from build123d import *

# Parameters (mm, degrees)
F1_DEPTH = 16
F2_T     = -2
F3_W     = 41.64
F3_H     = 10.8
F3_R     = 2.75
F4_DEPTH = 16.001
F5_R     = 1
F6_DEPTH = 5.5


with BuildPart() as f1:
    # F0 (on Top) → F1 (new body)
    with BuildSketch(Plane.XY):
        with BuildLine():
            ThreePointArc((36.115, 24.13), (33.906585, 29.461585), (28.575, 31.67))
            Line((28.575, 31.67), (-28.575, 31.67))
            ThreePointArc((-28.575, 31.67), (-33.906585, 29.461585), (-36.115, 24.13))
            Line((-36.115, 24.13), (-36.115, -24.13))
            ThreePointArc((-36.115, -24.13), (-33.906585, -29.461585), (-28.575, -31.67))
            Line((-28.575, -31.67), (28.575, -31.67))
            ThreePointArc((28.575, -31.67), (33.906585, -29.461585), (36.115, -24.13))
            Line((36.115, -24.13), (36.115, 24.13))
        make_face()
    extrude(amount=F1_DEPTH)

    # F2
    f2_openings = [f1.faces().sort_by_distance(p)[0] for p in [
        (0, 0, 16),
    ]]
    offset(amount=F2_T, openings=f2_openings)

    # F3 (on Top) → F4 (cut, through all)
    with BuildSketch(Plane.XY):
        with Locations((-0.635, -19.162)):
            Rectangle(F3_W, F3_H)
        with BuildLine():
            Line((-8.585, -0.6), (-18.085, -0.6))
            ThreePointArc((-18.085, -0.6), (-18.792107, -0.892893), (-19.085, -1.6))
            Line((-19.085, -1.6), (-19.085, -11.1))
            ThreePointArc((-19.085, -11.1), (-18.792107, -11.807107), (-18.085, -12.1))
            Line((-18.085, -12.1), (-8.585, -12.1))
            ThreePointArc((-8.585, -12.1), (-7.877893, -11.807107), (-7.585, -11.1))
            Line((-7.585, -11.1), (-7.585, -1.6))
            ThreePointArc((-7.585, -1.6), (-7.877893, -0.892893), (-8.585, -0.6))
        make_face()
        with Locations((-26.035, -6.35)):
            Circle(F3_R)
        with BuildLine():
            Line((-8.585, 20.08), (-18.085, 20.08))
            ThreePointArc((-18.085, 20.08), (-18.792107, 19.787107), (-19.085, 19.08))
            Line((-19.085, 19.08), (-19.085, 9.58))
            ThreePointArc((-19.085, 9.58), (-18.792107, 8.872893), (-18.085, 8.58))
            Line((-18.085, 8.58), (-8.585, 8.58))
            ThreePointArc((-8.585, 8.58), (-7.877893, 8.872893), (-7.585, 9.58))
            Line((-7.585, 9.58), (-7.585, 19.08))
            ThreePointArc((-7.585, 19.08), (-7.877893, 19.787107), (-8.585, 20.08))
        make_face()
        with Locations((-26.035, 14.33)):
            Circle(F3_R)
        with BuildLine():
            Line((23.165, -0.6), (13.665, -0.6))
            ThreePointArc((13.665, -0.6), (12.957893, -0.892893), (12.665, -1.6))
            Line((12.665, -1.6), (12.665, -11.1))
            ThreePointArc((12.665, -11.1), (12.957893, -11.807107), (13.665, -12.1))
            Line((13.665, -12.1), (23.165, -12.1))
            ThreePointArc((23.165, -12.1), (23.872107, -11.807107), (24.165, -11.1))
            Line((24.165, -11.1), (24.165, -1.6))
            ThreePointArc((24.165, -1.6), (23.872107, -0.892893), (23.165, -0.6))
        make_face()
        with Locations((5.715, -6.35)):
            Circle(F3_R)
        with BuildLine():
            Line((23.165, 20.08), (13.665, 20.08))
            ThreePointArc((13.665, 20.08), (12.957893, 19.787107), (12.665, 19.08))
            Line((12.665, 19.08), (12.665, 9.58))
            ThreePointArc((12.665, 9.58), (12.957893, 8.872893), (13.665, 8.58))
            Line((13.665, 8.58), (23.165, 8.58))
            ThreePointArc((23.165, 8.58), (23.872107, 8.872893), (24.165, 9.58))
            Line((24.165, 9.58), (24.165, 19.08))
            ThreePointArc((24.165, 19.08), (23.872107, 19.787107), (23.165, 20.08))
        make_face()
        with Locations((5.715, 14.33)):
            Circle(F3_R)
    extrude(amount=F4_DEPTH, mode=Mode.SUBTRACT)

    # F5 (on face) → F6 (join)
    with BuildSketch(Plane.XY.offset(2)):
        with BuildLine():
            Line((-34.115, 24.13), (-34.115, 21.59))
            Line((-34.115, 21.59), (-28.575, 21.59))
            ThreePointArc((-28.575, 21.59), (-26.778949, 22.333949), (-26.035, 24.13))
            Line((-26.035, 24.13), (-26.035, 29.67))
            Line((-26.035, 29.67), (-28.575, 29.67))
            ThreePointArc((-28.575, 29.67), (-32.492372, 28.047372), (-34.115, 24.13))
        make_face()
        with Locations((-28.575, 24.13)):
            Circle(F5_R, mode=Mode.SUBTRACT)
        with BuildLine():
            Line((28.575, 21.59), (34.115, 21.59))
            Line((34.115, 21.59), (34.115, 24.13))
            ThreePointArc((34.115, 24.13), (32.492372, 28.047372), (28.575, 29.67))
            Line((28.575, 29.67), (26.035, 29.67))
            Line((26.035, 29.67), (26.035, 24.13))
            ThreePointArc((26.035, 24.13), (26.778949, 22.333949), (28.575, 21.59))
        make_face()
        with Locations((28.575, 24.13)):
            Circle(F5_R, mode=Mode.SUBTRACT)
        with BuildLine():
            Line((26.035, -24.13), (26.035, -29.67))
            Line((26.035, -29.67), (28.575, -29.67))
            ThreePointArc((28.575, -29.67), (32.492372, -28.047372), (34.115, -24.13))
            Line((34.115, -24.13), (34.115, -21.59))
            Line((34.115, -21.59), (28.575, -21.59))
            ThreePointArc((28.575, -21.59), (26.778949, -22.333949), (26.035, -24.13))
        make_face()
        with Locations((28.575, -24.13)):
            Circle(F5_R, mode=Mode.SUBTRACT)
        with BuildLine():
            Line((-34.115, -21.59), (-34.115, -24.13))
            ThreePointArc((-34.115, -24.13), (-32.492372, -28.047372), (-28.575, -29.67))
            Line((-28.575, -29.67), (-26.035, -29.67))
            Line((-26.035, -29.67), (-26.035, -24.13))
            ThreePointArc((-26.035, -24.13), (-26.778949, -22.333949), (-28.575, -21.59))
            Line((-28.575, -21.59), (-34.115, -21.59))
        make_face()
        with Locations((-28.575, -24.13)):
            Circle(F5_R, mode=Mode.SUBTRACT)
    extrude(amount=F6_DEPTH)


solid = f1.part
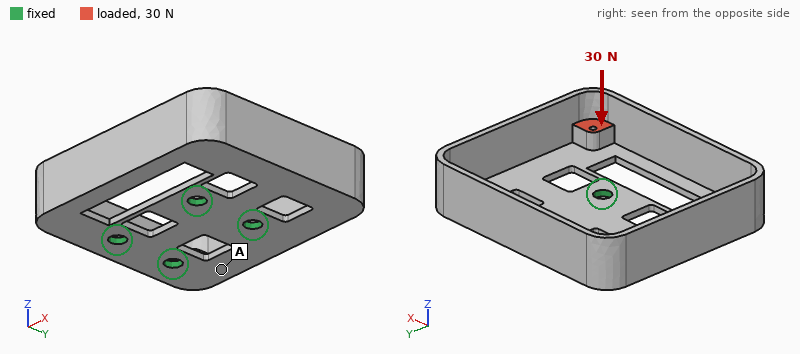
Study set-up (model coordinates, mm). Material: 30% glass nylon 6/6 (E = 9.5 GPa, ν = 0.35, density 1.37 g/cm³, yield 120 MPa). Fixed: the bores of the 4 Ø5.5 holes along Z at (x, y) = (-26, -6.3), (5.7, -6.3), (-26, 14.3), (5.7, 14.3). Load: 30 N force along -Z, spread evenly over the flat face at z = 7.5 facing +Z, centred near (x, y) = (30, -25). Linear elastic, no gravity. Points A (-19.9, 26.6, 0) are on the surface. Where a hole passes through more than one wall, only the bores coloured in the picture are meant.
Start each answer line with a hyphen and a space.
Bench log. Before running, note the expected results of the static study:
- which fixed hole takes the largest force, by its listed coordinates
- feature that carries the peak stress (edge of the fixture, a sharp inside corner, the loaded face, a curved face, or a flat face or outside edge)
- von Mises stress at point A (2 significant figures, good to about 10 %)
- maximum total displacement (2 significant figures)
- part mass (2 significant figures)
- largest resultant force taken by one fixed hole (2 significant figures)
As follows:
- (5.7, -6.3)
- a curved face
- 3.2 MPa
- 1.1 mm
- 21 g
- 30 N
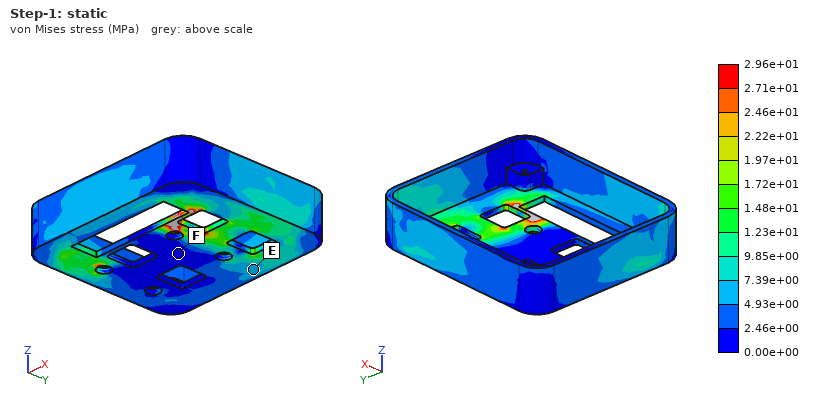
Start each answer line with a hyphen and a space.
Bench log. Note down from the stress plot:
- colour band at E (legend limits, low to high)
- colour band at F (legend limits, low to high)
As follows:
- 4.93e+00 to 7.39e+00 MPa
- 0.00e+00 to 2.46e+00 MPa
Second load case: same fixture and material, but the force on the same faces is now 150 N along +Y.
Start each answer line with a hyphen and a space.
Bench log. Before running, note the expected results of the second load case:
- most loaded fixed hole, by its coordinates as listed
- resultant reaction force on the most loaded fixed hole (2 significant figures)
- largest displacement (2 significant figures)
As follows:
- (5.7, 14.3)
- 140 N
- 0.90 mm
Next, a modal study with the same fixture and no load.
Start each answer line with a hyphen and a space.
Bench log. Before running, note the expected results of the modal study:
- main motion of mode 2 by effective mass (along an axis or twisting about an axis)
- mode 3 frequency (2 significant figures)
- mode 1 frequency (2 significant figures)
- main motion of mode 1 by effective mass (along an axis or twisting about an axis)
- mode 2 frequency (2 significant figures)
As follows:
- along Z
- 1700 Hz
- 460 Hz
- along Z
- 910 Hz
